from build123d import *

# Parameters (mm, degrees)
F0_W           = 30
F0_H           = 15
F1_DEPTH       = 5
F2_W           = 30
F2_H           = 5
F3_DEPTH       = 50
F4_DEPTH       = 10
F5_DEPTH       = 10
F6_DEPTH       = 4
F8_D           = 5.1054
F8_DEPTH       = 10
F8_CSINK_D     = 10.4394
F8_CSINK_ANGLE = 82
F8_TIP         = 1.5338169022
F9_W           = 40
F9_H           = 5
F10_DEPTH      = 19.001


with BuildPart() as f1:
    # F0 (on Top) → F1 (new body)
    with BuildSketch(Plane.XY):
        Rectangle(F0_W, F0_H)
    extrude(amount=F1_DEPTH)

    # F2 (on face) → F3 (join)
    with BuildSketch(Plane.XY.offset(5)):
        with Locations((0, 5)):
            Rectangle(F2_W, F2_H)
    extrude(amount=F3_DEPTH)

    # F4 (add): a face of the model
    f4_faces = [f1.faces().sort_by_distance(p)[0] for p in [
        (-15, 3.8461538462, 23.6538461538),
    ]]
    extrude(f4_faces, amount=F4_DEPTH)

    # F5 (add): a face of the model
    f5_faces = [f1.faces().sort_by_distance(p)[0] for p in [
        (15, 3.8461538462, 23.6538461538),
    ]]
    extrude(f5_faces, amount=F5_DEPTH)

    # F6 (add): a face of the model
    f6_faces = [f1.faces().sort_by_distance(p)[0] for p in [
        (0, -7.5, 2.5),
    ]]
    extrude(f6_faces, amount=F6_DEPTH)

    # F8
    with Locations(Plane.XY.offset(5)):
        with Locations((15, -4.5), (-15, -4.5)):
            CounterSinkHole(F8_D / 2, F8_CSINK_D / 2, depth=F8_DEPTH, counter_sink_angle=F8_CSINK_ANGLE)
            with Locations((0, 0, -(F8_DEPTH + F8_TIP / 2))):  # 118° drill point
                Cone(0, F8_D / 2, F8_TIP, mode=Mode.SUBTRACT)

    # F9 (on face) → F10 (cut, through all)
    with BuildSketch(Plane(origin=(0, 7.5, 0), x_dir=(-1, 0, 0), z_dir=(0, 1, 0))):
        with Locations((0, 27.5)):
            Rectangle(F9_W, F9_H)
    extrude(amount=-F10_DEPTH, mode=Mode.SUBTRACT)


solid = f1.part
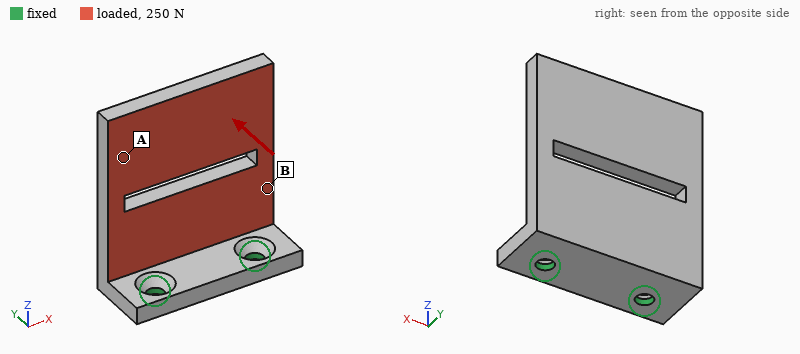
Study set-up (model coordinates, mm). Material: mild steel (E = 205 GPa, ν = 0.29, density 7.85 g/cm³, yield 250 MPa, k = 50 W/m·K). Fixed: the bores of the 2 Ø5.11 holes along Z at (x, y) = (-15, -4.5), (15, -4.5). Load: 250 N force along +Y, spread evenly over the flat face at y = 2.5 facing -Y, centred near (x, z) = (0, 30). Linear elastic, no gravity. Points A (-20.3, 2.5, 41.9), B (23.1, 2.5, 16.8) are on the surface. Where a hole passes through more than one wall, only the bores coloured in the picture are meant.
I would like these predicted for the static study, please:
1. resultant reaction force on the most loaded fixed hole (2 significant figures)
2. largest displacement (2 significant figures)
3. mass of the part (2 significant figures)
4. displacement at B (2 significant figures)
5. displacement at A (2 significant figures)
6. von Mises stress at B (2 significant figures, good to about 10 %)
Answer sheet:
140 N
0.14 mm
120 g
0.024 mm
0.096 mm
29 MPa
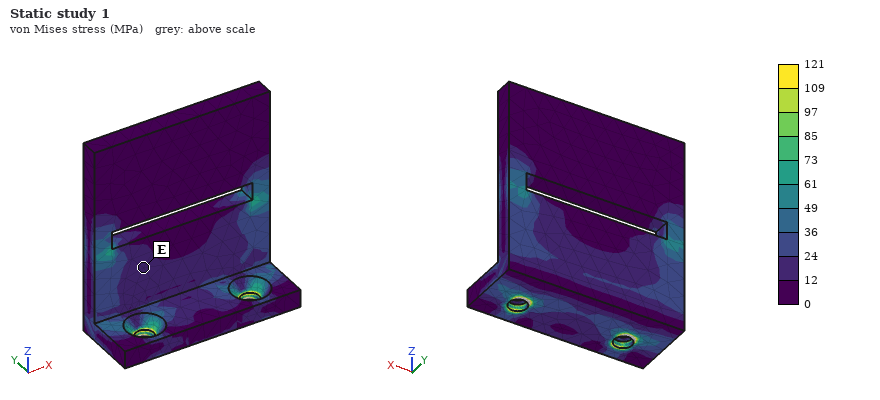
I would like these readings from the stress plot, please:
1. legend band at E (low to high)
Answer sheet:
12 to 24 MPa
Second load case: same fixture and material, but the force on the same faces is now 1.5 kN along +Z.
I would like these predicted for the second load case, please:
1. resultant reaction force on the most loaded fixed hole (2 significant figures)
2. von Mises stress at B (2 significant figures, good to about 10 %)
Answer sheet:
750 N
34 MPa
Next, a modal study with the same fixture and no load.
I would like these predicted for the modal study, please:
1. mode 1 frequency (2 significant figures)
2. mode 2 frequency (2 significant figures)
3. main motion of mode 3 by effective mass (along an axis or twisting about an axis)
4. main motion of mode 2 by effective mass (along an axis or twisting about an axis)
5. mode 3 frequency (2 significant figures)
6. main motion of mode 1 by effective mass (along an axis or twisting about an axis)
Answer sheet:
860 Hz
2700 Hz
along X
along X
3800 Hz
along Y
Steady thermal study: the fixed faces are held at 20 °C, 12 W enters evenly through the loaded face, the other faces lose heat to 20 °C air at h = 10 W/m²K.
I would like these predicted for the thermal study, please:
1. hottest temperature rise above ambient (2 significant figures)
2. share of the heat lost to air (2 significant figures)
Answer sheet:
59 K
13 %
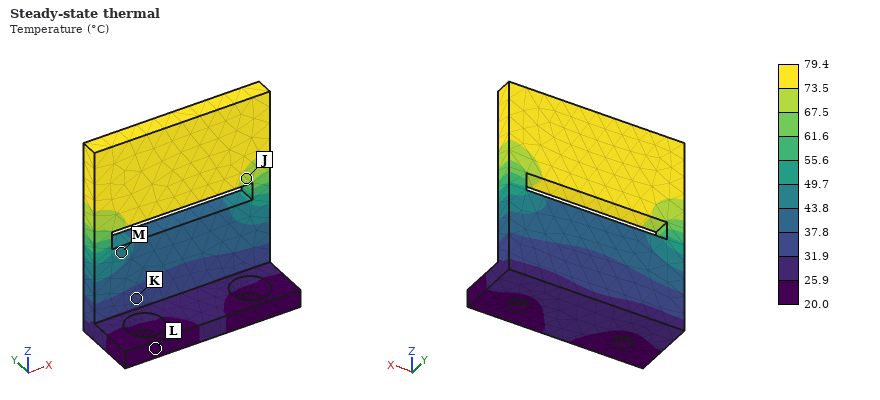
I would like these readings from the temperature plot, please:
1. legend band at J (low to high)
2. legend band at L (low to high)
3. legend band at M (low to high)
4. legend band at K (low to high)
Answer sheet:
67.5 to 73.5 °C
20.0 to 25.9 °C
43.8 to 49.7 °C
31.9 to 37.8 °C
